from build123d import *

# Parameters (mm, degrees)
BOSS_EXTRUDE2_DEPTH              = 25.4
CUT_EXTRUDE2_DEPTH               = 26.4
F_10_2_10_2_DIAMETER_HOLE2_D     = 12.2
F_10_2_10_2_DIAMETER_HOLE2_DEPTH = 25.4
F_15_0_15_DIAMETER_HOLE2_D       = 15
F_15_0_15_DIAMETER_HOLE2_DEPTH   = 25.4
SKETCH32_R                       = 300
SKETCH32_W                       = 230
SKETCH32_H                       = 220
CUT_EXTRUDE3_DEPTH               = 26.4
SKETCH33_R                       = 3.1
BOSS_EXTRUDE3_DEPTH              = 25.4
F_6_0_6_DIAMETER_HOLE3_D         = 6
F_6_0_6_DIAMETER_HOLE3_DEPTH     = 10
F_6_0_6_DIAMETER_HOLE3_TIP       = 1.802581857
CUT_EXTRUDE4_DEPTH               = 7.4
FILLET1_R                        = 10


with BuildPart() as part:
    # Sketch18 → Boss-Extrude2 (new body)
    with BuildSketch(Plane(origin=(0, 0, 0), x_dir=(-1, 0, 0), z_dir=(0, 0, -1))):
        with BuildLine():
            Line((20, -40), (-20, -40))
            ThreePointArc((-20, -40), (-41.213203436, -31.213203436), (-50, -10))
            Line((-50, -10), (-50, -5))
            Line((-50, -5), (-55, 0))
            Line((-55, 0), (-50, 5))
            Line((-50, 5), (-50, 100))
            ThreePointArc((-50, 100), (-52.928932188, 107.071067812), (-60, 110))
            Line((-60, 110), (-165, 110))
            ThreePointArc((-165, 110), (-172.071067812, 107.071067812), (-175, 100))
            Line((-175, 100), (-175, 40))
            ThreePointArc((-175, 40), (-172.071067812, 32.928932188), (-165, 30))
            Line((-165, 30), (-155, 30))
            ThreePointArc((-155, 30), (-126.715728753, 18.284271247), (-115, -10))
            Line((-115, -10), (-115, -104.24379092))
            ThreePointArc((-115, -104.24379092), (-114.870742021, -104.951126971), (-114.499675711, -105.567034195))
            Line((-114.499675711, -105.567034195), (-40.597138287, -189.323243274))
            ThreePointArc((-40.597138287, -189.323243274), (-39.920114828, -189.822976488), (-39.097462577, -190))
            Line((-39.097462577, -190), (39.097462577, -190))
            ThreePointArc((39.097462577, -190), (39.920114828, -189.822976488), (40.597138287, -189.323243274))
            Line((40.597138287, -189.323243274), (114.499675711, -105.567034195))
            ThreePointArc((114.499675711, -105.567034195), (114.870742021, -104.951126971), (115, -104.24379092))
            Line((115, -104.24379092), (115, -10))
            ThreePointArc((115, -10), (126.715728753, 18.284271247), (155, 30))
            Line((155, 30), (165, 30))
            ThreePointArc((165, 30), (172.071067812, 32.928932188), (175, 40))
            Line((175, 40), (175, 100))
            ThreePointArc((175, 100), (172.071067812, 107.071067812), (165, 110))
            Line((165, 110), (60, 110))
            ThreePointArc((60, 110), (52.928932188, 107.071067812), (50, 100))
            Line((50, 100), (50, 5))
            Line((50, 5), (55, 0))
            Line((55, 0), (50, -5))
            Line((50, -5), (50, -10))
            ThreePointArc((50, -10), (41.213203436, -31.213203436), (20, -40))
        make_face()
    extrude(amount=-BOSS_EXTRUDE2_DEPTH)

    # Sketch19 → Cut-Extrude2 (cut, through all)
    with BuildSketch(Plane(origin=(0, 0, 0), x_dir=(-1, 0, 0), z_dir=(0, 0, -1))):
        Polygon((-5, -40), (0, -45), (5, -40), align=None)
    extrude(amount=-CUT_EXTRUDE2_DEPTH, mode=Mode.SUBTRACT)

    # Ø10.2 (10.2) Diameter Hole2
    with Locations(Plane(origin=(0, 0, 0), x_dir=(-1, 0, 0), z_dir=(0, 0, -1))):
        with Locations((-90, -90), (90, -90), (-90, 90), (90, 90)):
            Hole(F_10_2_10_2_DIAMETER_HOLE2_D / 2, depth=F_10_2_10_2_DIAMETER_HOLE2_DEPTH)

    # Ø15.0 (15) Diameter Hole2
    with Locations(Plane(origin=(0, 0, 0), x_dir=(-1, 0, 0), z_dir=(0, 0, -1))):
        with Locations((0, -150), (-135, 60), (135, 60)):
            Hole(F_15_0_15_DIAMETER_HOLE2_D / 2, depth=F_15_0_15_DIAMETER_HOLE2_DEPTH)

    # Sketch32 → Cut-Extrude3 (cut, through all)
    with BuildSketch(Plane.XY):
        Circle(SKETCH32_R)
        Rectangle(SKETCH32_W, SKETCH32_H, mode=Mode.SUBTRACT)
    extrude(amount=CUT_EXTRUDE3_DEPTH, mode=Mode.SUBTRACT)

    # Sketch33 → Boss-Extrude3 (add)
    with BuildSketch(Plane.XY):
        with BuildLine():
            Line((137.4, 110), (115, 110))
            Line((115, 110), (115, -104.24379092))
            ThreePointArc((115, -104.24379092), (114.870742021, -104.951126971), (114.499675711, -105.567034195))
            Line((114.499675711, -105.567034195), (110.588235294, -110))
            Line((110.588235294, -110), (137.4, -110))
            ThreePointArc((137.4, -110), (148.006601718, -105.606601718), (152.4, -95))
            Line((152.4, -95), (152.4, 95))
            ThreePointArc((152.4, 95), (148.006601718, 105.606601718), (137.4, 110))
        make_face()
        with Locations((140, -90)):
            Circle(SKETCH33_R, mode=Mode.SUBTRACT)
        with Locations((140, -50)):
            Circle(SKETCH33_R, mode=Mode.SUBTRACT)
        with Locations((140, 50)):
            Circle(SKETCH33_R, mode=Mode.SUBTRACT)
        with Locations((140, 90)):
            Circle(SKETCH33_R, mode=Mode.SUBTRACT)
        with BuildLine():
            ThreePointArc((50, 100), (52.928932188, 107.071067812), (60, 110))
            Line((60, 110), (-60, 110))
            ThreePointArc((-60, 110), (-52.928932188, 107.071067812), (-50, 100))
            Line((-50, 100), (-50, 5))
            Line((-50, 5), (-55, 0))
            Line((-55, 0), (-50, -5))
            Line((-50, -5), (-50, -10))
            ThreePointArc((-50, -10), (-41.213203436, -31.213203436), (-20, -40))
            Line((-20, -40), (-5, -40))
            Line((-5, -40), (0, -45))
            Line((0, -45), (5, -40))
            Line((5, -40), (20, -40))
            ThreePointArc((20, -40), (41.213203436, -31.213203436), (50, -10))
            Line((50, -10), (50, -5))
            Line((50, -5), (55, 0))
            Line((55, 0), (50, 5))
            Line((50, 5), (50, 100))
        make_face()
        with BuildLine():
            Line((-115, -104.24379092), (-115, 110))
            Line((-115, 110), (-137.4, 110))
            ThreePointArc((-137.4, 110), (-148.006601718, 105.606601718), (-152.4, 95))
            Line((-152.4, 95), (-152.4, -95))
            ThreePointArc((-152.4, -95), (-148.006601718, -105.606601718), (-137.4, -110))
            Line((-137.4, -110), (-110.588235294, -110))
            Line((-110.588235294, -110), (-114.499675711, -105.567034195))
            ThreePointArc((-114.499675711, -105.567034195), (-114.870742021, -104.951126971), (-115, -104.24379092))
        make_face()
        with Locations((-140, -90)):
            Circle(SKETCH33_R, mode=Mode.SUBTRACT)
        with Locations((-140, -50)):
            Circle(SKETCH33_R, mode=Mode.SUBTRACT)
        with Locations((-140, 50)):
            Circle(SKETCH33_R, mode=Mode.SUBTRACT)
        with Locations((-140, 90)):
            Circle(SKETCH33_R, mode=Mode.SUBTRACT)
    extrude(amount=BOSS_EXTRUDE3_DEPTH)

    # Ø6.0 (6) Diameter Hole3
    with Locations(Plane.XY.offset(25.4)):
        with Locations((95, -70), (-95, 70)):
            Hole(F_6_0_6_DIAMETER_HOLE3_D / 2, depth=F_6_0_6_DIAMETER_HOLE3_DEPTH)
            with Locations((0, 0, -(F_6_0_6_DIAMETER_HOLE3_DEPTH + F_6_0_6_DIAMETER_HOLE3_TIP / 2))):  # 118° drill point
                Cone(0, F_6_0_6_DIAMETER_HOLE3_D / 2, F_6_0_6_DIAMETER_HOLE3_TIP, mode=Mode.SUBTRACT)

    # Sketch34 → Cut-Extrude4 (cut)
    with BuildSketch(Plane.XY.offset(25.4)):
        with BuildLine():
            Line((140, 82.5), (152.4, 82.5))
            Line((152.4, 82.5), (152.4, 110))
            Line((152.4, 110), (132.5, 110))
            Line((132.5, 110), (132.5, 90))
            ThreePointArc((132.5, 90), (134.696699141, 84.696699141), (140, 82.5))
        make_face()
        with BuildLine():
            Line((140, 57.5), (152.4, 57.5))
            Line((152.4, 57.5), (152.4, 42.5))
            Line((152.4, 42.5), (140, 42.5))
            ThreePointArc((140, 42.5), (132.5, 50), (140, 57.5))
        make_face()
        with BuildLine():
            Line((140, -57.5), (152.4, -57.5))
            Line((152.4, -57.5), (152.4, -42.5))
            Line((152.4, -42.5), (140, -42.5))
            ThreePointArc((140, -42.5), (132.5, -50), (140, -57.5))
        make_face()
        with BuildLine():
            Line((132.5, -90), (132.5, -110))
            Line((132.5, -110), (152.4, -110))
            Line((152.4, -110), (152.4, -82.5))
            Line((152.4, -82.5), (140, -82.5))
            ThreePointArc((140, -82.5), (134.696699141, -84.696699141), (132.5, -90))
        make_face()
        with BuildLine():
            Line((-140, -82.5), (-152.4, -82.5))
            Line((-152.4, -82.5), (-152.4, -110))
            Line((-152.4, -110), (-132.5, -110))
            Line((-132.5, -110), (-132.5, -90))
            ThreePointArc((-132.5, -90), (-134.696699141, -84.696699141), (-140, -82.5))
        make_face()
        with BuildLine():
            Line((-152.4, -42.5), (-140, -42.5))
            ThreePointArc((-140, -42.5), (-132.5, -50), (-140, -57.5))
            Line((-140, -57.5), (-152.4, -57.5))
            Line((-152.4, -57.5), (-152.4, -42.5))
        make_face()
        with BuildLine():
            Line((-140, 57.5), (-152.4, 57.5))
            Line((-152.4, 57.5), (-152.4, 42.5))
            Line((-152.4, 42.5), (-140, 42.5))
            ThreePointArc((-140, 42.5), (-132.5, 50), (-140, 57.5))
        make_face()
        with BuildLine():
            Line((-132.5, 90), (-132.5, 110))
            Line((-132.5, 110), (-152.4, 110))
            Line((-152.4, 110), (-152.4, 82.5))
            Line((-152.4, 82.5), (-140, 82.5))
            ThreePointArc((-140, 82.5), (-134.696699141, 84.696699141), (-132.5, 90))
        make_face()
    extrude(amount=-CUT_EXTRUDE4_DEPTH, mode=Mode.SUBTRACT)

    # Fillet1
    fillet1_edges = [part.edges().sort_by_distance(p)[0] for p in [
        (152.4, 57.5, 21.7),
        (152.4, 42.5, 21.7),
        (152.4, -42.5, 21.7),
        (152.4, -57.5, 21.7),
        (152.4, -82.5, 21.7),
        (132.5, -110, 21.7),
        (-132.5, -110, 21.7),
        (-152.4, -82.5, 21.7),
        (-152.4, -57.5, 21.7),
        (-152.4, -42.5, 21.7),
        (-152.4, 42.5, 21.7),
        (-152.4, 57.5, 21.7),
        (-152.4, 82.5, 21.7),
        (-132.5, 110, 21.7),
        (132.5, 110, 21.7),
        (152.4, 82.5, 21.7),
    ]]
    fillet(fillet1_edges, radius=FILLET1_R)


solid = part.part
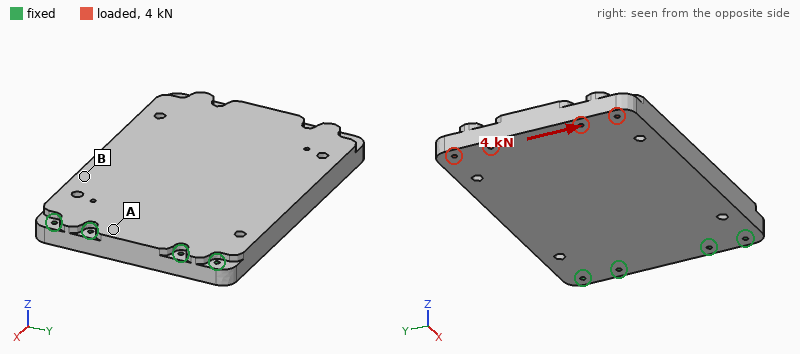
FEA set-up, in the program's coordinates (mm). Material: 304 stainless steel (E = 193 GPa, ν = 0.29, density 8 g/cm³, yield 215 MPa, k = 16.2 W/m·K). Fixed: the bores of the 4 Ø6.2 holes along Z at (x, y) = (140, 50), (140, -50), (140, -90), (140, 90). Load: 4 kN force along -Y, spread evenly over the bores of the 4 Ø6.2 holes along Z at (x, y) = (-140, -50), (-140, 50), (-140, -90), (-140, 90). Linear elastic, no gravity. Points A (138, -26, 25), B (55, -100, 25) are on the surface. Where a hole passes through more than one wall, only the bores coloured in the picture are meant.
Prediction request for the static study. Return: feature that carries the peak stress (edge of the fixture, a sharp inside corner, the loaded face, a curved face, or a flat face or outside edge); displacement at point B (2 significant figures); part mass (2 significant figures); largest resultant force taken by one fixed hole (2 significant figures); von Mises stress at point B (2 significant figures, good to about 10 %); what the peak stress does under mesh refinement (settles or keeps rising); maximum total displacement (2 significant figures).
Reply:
edge of the fixture
5.0 µm
13 kg
4.9 kN
3.1 MPa
keeps rising
16 µm
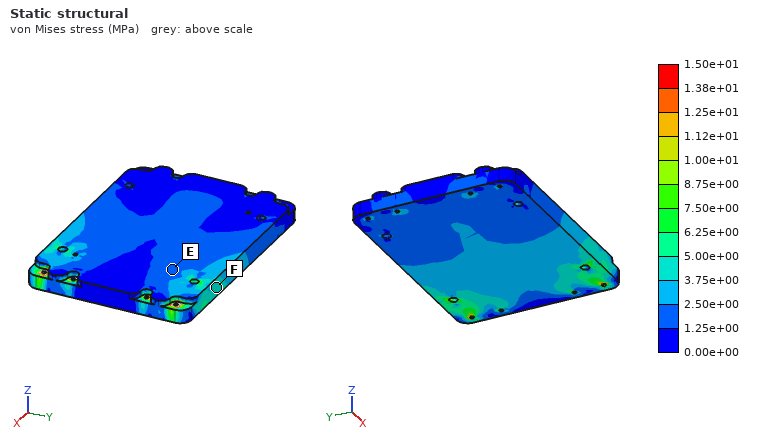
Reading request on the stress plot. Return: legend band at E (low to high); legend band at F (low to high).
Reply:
1.25e+00 to 2.50e+00 MPa
3.75e+00 to 5.00e+00 MPa
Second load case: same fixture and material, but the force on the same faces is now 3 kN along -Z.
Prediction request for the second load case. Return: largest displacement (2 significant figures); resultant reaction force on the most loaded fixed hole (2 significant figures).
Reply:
0.61 mm
1.8 kN
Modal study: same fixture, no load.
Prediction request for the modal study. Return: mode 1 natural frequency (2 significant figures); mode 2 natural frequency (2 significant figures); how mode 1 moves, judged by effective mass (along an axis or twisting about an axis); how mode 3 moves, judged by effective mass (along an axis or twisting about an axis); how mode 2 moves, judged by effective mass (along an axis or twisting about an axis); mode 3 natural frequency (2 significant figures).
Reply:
190 Hz
670 Hz
along Z
along Z
twisting about X
1200 Hz
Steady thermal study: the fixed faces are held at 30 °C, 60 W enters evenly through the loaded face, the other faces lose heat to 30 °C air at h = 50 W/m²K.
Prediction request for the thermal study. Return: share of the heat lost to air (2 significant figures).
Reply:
99 %
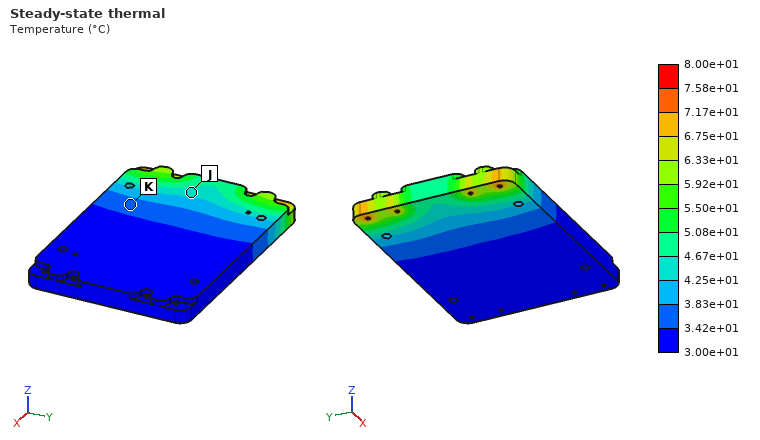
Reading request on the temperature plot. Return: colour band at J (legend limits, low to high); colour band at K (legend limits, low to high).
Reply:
4.25e+01 to 4.67e+01 °C
3.42e+01 to 3.83e+01 °C
